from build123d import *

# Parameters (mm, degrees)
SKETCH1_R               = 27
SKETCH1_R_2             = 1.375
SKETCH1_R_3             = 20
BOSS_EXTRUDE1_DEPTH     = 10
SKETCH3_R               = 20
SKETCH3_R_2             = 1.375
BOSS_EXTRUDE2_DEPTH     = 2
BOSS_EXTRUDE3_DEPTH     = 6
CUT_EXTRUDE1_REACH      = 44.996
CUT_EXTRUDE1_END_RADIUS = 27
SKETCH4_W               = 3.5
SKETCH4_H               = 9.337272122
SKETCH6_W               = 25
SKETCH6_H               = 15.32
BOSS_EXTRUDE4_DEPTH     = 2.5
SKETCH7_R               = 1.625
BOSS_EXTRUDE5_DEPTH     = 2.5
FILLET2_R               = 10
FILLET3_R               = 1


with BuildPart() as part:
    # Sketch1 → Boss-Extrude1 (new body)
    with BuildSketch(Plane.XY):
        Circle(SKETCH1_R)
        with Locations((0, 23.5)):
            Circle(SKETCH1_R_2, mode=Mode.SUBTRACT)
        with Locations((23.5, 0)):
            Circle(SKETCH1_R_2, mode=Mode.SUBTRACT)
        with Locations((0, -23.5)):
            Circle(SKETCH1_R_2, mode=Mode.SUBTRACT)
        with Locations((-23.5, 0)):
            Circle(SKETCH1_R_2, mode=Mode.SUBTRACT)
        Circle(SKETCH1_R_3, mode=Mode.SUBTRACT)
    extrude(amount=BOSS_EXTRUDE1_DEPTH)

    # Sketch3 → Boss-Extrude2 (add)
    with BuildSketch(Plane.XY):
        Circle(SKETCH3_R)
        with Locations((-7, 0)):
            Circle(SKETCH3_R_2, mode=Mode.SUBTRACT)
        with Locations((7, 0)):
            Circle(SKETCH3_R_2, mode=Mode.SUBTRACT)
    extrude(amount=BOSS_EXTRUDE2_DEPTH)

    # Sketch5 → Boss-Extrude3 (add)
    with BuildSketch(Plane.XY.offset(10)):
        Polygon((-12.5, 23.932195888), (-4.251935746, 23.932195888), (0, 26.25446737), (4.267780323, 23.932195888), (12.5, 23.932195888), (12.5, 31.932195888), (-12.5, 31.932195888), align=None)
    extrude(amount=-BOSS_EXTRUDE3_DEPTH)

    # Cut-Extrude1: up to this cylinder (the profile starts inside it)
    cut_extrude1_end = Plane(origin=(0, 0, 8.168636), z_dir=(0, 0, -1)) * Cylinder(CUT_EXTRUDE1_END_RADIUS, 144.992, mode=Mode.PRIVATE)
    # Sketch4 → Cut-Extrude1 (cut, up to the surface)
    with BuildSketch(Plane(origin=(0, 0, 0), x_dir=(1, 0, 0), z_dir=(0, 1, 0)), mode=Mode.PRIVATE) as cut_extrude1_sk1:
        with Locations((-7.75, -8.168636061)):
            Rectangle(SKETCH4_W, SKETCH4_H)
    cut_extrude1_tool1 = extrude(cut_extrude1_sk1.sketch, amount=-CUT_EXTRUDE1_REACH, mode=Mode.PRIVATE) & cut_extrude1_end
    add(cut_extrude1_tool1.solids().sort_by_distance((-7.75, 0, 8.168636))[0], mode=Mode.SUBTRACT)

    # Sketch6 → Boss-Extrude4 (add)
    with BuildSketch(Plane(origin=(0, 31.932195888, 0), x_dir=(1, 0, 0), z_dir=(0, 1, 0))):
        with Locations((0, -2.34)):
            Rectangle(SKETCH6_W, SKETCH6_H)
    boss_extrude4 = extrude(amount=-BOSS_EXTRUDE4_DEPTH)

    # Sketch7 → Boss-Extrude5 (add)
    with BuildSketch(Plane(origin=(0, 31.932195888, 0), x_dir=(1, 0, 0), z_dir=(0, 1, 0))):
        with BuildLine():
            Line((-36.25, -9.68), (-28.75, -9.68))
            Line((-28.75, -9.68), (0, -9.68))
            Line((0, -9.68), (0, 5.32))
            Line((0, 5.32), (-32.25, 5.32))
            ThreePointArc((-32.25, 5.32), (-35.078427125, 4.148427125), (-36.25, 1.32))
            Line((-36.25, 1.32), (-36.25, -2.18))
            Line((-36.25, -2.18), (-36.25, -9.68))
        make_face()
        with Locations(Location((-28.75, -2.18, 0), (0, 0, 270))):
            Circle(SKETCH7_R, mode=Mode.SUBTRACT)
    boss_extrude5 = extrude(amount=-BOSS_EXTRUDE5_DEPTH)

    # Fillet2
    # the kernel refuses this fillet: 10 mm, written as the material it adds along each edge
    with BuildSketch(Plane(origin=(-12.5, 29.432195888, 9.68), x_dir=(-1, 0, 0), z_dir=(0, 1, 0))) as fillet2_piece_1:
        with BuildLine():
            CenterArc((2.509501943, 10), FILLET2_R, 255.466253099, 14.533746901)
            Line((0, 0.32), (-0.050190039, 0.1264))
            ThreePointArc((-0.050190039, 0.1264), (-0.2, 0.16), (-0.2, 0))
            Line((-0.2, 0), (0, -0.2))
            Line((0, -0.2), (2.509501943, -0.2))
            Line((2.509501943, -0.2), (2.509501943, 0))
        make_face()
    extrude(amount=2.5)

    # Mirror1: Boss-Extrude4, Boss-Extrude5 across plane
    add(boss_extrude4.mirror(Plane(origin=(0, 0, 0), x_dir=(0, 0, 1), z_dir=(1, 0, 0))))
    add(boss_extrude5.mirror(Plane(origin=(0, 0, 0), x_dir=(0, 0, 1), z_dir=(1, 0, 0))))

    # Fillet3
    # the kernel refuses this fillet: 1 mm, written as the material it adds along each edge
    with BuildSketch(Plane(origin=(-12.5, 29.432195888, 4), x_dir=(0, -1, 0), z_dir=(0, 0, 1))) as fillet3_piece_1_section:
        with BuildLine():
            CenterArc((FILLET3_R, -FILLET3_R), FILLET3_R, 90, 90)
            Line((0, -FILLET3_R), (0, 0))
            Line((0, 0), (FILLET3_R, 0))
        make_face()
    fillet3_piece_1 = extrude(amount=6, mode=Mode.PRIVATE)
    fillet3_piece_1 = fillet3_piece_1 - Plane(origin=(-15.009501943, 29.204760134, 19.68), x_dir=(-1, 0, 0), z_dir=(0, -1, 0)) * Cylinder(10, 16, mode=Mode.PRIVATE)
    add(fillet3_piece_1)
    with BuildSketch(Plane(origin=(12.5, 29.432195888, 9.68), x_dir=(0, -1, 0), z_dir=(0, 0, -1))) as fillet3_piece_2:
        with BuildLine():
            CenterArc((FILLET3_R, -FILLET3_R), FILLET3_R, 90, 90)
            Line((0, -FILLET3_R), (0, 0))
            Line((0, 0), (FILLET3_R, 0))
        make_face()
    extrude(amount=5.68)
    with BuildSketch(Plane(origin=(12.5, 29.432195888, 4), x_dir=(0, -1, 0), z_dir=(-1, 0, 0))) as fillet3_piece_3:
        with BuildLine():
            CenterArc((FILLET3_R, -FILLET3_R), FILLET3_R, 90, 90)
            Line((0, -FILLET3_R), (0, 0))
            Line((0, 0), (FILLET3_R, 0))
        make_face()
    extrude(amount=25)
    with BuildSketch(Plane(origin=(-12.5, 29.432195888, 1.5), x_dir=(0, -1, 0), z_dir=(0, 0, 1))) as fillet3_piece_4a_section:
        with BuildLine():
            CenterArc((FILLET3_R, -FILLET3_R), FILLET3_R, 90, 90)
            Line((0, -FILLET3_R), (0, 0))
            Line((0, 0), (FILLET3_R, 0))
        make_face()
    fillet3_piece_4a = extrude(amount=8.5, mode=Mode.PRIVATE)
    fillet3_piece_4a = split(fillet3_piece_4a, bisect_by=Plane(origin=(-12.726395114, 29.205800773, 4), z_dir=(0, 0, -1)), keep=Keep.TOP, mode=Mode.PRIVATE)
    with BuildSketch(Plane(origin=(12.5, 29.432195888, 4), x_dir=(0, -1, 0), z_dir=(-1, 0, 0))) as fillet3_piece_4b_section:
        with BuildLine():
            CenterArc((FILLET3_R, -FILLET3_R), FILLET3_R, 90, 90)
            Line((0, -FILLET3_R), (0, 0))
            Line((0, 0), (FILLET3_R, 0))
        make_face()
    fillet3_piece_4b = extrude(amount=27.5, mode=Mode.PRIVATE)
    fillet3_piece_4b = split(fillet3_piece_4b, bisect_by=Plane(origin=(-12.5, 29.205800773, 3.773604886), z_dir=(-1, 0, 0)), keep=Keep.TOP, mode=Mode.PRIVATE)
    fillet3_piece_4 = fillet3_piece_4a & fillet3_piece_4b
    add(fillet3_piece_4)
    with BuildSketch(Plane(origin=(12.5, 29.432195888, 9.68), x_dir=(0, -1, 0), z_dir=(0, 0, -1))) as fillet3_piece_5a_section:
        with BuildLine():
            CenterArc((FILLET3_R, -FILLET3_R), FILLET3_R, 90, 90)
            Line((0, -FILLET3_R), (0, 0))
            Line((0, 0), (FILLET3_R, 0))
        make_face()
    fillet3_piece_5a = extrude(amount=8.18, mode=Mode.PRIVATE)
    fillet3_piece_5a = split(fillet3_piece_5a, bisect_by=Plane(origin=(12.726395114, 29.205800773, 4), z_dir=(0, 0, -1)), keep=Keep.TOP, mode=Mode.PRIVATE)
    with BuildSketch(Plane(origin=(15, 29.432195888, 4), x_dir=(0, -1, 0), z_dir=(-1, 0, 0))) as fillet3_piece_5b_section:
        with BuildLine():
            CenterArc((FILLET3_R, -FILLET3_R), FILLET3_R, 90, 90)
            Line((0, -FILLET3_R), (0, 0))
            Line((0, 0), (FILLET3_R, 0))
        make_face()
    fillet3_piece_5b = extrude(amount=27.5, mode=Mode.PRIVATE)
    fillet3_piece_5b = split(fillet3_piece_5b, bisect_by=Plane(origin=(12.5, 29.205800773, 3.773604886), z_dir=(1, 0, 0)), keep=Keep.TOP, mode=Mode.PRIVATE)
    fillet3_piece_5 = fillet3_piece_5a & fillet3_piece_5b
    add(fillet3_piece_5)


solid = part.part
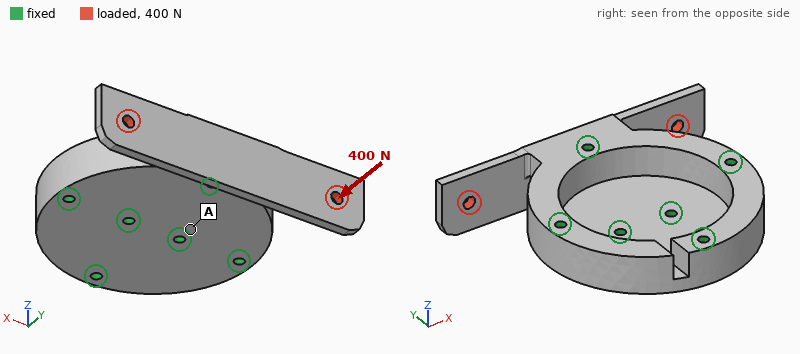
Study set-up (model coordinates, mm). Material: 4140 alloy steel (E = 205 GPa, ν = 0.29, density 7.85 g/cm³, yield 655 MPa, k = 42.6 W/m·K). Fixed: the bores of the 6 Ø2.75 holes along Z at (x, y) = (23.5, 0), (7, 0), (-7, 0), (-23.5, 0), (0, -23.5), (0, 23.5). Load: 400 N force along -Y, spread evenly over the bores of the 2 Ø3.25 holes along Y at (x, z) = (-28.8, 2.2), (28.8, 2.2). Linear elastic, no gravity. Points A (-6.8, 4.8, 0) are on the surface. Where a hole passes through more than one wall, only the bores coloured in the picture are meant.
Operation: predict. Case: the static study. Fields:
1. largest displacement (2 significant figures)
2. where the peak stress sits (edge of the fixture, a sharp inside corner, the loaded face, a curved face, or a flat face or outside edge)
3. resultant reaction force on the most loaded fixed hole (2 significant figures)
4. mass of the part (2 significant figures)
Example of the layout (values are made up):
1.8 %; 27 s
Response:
0.18 mm; a curved face; 140 N; 120 g
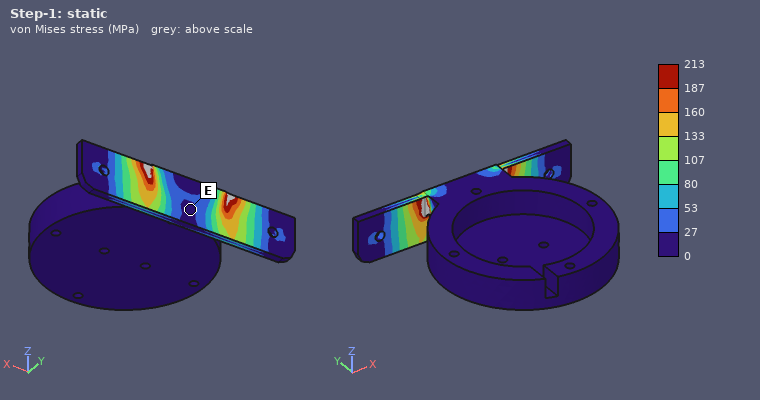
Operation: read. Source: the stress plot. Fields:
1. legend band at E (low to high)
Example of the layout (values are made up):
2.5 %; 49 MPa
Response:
0 to 27 MPa
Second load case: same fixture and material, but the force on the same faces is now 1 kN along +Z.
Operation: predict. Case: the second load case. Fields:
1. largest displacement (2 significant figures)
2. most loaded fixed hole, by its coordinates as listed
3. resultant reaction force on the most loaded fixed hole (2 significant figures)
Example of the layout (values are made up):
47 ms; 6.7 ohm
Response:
34 µm; (0, 23.5); 1.0 kN
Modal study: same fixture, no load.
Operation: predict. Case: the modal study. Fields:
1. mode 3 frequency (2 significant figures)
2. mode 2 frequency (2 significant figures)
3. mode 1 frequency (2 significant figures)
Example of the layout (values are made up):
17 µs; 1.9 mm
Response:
6500 Hz; 3100 Hz; 3000 Hz
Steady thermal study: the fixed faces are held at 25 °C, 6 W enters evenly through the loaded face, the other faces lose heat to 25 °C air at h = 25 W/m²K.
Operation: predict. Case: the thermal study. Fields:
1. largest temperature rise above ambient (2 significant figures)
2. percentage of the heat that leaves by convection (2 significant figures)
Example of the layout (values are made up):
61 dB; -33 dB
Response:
43 K; 26 %
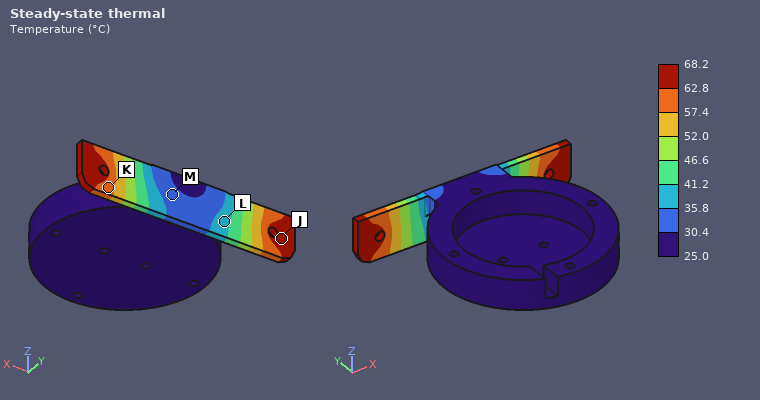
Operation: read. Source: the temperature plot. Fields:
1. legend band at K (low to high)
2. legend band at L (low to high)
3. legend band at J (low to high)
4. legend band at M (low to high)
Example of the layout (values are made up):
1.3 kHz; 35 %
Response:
57.4 to 62.8 °C; 35.8 to 41.2 °C; 62.8 to 68.2 °C; 30.4 to 35.8 °C
